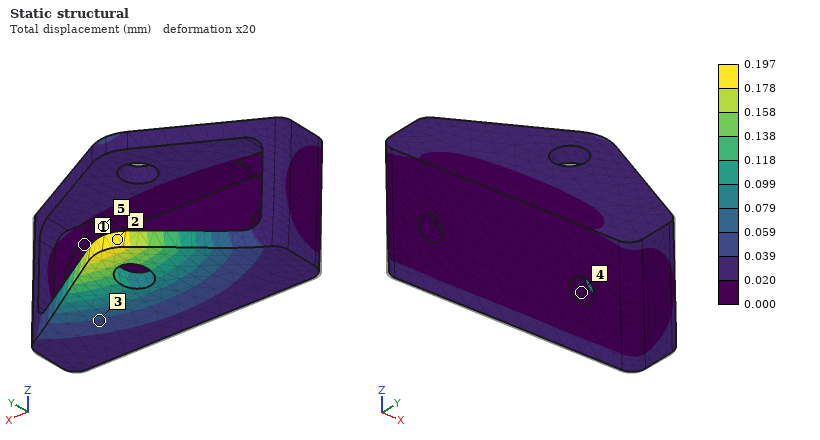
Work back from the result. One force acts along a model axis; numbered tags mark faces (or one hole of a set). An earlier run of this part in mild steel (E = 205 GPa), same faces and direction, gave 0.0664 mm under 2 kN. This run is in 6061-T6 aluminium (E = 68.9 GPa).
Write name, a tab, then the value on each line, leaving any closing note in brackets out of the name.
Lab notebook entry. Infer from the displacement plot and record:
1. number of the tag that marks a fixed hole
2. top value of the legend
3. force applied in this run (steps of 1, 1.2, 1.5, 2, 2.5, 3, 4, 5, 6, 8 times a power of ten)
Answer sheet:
number of the tag that marks a fixed hole	4
top value of the legend	0.197 mm
force applied in this run	2 kN
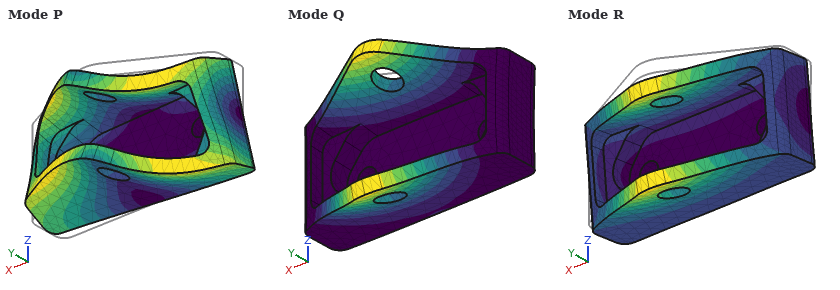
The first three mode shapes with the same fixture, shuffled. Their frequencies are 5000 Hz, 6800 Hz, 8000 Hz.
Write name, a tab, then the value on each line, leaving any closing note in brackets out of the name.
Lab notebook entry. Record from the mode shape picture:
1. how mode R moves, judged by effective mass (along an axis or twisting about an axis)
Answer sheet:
how mode R moves, judged by effective mass	along Z
